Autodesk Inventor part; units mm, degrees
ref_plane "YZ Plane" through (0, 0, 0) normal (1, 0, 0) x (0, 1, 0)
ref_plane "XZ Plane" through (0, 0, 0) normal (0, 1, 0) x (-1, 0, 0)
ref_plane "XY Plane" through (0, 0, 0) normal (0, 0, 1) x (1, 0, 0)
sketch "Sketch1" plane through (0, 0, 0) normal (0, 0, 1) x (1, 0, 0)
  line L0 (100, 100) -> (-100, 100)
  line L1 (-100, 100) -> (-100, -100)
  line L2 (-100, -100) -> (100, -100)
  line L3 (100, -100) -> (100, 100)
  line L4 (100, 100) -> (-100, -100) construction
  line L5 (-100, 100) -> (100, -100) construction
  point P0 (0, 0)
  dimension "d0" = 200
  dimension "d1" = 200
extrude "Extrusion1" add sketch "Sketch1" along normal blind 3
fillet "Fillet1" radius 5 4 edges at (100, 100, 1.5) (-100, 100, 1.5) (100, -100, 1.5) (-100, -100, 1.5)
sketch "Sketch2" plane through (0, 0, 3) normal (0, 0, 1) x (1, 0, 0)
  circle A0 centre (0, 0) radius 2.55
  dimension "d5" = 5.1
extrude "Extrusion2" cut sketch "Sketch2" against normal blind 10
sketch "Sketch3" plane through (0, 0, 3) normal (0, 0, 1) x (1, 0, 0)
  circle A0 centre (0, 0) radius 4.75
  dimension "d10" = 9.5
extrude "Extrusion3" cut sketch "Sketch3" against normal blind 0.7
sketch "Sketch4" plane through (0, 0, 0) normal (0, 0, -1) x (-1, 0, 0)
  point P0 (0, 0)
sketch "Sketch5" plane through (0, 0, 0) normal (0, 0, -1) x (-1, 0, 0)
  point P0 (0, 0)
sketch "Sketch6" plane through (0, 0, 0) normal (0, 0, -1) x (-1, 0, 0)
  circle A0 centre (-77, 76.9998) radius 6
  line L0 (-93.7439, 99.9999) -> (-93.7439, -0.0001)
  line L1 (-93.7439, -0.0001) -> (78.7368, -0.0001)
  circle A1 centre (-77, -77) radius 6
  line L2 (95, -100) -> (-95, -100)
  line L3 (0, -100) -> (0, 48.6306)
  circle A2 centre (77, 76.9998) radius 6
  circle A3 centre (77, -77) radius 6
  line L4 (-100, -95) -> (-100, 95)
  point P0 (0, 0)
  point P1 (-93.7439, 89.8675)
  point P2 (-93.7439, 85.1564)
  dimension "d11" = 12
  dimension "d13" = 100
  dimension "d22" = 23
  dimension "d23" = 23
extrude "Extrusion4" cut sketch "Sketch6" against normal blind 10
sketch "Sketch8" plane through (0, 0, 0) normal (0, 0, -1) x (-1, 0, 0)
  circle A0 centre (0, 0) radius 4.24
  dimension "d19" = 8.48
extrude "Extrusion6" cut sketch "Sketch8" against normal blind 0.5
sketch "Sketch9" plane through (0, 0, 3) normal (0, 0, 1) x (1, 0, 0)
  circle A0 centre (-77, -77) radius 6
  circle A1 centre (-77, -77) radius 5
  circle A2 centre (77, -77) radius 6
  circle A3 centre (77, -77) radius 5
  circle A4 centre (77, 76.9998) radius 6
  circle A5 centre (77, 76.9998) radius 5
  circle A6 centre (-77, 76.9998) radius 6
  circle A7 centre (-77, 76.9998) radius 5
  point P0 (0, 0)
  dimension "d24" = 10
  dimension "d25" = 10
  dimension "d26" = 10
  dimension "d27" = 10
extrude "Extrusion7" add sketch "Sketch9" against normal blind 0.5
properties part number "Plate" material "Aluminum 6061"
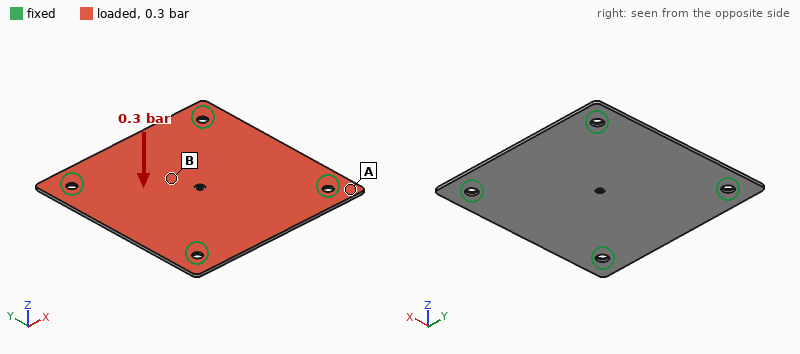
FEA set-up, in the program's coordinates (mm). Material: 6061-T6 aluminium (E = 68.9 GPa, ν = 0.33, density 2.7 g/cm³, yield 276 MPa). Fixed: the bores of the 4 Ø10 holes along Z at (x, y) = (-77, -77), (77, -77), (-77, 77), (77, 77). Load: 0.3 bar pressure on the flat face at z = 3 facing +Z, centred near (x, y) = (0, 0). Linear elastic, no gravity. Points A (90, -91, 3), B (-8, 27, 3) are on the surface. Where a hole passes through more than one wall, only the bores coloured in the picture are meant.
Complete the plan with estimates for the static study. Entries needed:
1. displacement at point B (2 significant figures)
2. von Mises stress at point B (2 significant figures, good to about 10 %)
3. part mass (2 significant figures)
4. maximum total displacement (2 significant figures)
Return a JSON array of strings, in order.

["0.75 mm", "23 MPa", "320 g", "0.83 mm"]
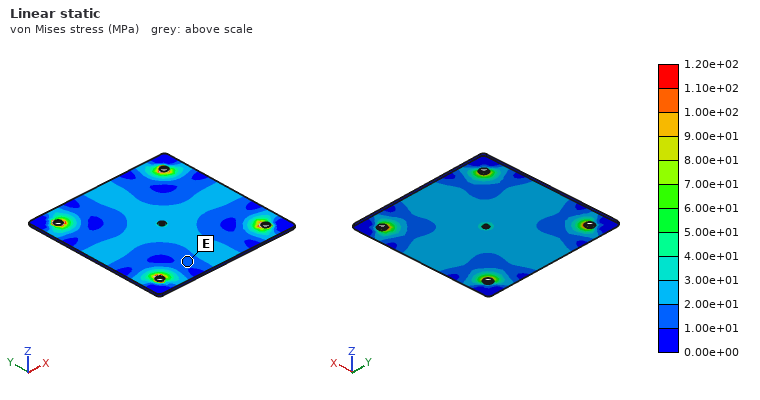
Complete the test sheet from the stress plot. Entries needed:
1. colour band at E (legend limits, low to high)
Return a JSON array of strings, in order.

["1.00e+01 to 2.00e+01 MPa"]
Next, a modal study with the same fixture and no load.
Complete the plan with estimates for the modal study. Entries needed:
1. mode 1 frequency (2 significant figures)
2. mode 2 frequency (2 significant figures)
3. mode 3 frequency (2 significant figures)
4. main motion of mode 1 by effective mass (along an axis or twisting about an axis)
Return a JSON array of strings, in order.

["410 Hz", "660 Hz", "660 Hz", "along Z"]
